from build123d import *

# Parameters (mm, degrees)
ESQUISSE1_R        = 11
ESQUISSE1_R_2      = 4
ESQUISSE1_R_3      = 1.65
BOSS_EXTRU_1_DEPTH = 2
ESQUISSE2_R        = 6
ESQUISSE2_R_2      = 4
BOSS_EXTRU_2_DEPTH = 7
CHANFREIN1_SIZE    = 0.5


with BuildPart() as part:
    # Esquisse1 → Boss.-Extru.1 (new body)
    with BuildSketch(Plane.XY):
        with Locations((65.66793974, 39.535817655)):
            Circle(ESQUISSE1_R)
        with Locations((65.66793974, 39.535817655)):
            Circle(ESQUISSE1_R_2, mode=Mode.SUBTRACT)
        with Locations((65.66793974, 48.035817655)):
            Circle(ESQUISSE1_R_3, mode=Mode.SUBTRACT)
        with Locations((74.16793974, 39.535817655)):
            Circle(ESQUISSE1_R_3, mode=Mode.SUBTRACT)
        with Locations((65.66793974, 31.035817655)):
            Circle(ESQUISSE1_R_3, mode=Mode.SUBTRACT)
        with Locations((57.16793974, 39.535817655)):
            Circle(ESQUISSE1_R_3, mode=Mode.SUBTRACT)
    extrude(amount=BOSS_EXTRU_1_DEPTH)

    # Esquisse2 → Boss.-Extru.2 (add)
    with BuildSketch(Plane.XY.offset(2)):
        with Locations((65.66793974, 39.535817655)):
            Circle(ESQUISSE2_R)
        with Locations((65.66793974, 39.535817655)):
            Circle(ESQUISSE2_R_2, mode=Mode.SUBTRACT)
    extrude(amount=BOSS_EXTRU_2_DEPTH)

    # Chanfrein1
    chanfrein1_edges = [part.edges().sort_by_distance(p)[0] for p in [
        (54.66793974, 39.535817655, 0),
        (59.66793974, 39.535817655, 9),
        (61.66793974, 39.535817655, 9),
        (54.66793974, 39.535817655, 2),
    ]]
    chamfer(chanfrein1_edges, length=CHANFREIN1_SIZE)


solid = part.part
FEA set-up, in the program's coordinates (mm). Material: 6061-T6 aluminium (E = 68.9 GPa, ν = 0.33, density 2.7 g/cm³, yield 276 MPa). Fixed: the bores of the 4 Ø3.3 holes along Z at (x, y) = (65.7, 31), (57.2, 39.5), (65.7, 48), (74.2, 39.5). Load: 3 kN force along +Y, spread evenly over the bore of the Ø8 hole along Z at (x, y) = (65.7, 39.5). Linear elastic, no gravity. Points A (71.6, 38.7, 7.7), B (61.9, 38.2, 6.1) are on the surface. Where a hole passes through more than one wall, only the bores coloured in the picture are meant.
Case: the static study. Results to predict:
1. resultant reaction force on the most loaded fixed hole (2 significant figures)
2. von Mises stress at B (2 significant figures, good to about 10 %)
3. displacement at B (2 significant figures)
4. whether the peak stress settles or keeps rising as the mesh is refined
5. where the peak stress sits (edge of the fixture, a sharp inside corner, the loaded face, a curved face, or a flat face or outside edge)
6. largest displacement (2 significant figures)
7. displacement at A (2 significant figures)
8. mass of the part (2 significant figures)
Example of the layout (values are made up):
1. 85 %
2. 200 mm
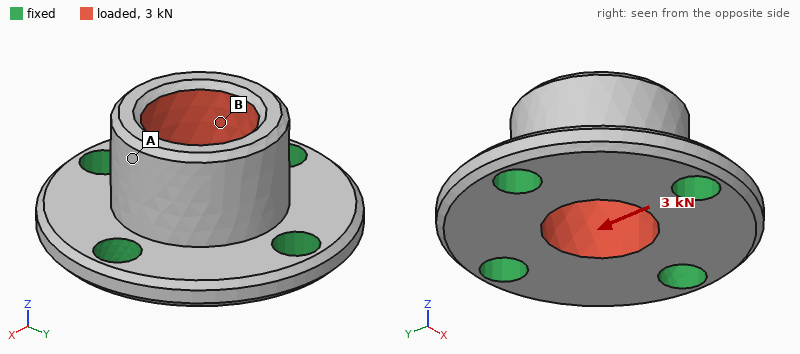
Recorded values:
1. 1.1 kN
2. 62 MPa
3. 15 µm
4. keeps rising
5. edge of the fixture
6. 22 µm
7. 16 µm
8. 2.7 g
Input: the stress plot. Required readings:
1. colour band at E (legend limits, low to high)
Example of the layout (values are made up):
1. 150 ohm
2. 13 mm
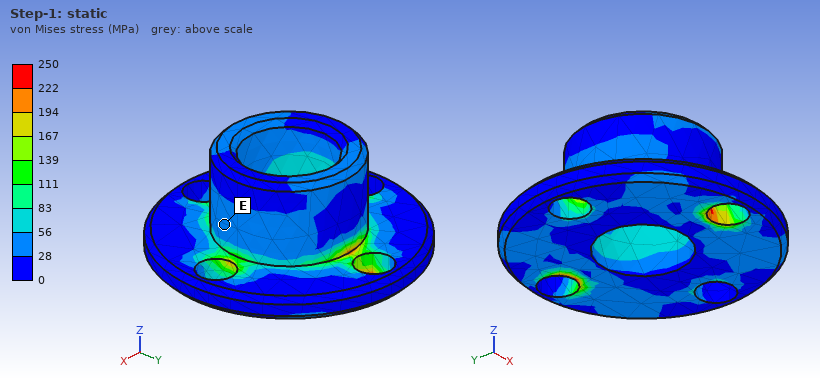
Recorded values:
1. 28 to 56 MPa
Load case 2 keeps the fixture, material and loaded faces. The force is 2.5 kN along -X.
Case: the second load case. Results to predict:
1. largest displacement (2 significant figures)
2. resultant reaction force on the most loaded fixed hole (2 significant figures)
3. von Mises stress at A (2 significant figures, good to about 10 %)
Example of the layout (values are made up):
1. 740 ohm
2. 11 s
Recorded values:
1. 19 µm
2. 920 N
3. 21 MPa
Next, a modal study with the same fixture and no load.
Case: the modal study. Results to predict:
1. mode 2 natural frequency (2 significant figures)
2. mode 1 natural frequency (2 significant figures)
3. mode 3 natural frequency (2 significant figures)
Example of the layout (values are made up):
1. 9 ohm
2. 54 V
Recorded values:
1. 52 kHz
2. 52 kHz
3. 59 kHz
